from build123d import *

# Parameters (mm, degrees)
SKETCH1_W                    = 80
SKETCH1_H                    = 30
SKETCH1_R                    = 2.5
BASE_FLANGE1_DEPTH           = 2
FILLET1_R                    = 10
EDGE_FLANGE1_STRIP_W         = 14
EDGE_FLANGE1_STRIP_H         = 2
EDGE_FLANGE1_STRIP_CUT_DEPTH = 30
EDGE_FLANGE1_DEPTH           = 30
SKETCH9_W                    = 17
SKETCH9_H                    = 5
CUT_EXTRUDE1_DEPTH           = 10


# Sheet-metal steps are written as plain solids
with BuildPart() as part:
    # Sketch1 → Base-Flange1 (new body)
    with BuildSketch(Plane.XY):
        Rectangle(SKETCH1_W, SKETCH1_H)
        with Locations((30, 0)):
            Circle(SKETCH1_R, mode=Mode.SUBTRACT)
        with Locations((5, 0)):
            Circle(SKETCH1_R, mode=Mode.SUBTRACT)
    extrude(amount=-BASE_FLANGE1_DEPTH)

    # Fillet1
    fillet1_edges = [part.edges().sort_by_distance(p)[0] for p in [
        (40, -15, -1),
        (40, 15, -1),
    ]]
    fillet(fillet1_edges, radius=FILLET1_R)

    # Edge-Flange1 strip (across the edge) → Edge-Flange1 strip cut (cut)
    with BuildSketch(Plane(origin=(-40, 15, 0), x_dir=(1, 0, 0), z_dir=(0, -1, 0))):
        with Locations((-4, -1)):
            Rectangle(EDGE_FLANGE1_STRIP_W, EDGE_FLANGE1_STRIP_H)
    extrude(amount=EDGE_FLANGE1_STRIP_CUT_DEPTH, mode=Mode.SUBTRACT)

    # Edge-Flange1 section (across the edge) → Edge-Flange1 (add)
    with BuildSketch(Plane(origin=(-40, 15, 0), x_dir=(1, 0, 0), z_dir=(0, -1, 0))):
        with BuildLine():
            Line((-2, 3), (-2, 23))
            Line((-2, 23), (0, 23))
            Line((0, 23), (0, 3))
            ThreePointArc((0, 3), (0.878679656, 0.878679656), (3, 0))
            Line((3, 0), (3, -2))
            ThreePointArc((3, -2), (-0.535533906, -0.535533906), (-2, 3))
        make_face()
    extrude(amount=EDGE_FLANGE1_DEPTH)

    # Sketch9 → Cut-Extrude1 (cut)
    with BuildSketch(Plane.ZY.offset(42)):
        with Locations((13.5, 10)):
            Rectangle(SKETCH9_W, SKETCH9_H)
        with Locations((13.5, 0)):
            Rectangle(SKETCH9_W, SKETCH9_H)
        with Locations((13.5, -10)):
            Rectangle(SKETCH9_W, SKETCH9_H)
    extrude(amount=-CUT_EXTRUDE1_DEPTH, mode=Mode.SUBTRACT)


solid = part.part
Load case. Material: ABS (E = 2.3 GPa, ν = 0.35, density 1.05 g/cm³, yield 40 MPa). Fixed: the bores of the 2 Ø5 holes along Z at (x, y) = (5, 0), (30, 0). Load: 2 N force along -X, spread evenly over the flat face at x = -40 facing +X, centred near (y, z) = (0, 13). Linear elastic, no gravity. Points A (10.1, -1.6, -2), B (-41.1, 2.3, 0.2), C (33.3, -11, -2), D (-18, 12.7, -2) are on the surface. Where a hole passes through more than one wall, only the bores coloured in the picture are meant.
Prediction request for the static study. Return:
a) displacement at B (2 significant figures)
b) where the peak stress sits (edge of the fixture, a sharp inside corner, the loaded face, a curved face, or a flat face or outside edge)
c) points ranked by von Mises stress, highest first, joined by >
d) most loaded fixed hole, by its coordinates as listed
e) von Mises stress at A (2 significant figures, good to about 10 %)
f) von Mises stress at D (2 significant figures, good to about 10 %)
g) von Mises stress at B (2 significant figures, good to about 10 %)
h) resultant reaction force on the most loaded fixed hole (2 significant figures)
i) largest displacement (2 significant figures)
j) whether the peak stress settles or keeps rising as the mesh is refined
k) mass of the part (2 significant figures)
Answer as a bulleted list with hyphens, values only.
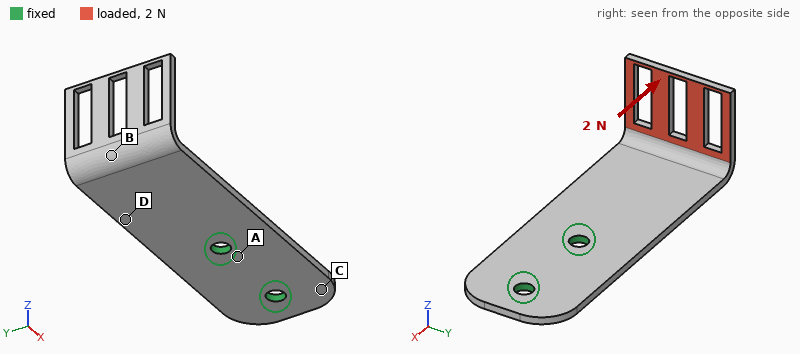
- 0.60 mm
- edge of the fixture
- D > B > A > C
- (5, 0)
- 0.32 MPa
- 1.3 MPa
- 0.94 MPa
- 1.6 N
- 0.95 mm
- keeps rising
- 5.8 g
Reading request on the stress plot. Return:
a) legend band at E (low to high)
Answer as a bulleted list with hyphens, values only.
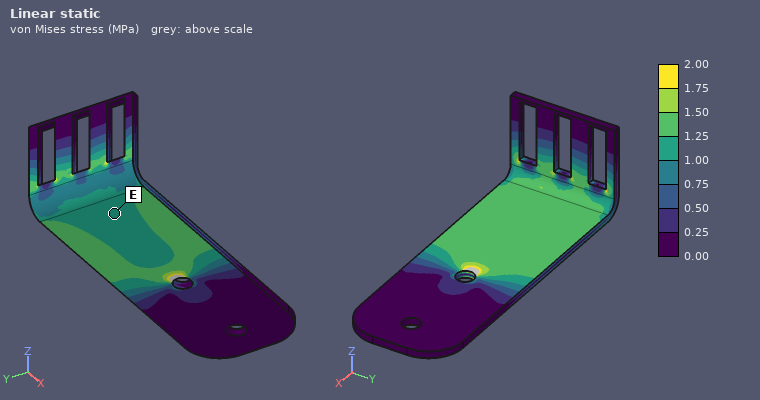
- 1.00 to 1.25 MPa
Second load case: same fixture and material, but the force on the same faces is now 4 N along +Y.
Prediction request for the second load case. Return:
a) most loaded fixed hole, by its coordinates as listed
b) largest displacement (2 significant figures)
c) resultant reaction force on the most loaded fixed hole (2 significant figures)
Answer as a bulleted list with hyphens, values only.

- (5, 0)
- 1.0 mm
- 9.5 N
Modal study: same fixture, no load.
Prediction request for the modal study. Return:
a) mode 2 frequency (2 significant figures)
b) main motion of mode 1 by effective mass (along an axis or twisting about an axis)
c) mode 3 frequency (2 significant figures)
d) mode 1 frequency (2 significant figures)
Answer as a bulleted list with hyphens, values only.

- 360 Hz
- along Z
- 590 Hz
- 150 Hz
